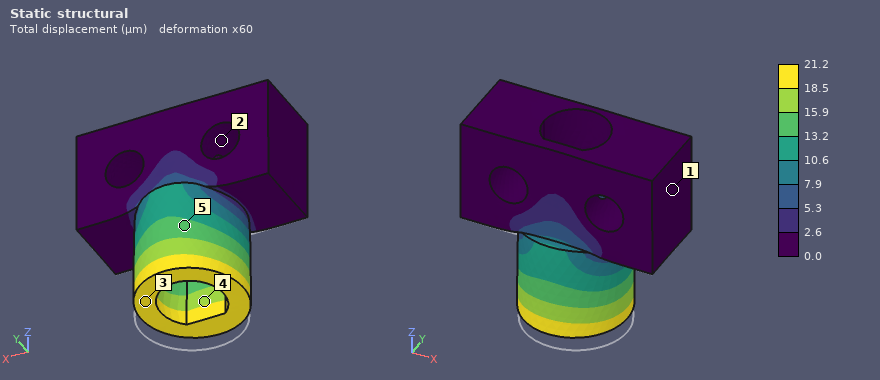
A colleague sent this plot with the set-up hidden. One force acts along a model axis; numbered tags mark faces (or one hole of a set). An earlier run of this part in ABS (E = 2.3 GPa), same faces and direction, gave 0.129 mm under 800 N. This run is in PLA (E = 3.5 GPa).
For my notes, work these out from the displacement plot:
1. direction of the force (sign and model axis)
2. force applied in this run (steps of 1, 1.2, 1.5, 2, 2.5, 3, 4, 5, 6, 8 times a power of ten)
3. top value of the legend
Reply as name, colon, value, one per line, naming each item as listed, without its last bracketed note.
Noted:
direction of the force: +Z
force applied in this run: 200 N
top value of the legend: 21.2 µm
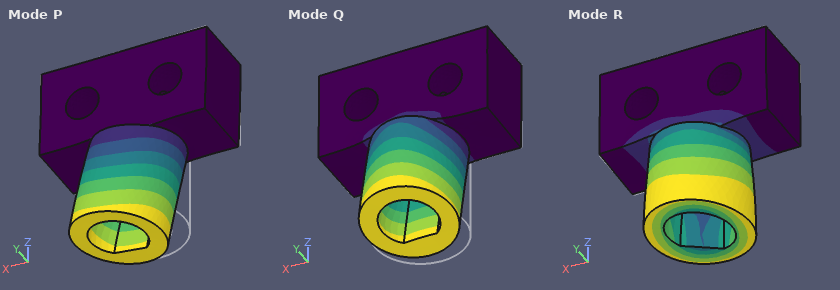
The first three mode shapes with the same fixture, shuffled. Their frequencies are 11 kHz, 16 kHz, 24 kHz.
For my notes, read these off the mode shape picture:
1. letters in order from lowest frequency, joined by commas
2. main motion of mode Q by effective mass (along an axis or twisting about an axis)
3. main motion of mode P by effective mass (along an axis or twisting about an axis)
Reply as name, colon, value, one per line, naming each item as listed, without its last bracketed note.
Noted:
letters in order from lowest frequency, joined by commas: Q, P, R
main motion of mode Q by effective mass: along Y
main motion of mode P by effective mass: along X
